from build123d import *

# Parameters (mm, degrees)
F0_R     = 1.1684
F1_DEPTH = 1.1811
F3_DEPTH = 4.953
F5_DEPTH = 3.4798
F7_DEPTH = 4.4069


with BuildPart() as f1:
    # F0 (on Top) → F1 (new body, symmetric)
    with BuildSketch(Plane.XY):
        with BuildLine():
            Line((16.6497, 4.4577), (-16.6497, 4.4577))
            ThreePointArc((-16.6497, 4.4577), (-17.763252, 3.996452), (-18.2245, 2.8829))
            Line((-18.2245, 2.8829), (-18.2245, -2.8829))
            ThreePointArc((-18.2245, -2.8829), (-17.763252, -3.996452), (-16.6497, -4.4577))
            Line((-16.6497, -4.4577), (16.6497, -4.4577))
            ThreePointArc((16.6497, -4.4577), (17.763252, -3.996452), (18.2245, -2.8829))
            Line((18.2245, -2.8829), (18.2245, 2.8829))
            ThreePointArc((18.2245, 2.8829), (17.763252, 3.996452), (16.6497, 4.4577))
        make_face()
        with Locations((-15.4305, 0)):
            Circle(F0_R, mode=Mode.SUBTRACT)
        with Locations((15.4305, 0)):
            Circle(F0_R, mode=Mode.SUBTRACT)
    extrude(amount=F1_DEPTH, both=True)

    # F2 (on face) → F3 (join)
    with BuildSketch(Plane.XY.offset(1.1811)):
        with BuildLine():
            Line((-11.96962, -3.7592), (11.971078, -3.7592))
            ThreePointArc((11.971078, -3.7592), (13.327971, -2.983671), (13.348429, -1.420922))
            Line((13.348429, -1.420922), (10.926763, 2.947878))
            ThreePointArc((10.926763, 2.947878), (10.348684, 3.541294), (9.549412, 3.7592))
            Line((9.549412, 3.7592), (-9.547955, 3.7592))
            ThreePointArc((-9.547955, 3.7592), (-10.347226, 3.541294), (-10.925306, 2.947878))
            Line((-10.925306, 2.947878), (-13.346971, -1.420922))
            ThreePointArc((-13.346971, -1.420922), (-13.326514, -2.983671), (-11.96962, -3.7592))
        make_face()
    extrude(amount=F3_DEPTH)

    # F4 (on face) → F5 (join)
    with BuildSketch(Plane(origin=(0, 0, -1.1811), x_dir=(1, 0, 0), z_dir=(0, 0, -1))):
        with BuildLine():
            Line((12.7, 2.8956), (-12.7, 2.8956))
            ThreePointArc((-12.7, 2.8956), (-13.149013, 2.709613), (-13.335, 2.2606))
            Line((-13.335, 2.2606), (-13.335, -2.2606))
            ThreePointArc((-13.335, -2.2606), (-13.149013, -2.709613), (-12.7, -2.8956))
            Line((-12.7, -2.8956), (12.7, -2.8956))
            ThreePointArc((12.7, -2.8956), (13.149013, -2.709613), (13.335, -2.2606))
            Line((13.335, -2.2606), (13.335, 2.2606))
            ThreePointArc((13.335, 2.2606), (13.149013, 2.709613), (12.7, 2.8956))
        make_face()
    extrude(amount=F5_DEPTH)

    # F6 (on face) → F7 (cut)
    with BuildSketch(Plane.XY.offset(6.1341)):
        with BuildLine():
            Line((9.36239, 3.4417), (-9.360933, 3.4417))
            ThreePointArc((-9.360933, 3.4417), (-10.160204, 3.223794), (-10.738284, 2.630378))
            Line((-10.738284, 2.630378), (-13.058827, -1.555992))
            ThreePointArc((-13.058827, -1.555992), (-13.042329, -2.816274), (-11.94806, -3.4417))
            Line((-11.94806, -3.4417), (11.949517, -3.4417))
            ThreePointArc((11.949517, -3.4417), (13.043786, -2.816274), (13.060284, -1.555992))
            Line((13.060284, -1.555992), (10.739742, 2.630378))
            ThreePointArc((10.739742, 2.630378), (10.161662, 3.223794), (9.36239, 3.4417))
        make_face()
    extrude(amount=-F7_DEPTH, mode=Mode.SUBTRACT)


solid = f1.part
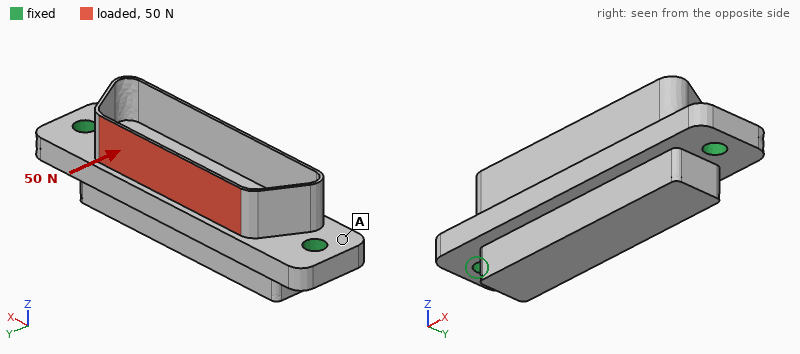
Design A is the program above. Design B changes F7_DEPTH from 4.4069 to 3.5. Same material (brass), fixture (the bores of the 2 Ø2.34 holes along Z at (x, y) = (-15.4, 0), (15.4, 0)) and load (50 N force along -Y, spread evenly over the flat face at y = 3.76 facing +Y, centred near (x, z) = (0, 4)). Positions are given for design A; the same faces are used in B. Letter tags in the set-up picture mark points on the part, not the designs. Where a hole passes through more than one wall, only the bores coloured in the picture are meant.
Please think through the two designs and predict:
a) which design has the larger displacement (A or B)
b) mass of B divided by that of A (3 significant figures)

A
1.10
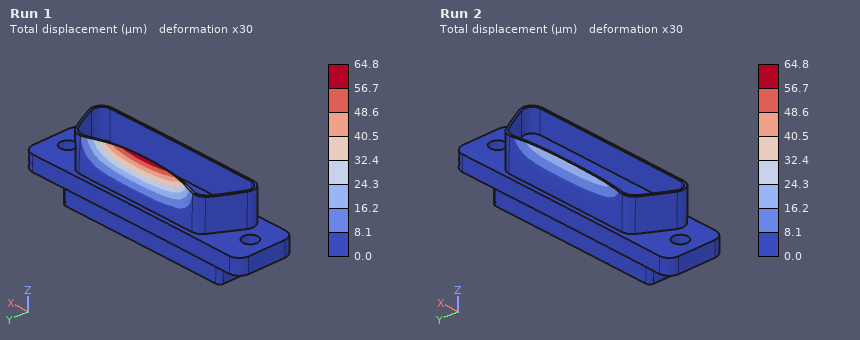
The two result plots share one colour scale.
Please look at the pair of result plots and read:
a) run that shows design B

Run 2
